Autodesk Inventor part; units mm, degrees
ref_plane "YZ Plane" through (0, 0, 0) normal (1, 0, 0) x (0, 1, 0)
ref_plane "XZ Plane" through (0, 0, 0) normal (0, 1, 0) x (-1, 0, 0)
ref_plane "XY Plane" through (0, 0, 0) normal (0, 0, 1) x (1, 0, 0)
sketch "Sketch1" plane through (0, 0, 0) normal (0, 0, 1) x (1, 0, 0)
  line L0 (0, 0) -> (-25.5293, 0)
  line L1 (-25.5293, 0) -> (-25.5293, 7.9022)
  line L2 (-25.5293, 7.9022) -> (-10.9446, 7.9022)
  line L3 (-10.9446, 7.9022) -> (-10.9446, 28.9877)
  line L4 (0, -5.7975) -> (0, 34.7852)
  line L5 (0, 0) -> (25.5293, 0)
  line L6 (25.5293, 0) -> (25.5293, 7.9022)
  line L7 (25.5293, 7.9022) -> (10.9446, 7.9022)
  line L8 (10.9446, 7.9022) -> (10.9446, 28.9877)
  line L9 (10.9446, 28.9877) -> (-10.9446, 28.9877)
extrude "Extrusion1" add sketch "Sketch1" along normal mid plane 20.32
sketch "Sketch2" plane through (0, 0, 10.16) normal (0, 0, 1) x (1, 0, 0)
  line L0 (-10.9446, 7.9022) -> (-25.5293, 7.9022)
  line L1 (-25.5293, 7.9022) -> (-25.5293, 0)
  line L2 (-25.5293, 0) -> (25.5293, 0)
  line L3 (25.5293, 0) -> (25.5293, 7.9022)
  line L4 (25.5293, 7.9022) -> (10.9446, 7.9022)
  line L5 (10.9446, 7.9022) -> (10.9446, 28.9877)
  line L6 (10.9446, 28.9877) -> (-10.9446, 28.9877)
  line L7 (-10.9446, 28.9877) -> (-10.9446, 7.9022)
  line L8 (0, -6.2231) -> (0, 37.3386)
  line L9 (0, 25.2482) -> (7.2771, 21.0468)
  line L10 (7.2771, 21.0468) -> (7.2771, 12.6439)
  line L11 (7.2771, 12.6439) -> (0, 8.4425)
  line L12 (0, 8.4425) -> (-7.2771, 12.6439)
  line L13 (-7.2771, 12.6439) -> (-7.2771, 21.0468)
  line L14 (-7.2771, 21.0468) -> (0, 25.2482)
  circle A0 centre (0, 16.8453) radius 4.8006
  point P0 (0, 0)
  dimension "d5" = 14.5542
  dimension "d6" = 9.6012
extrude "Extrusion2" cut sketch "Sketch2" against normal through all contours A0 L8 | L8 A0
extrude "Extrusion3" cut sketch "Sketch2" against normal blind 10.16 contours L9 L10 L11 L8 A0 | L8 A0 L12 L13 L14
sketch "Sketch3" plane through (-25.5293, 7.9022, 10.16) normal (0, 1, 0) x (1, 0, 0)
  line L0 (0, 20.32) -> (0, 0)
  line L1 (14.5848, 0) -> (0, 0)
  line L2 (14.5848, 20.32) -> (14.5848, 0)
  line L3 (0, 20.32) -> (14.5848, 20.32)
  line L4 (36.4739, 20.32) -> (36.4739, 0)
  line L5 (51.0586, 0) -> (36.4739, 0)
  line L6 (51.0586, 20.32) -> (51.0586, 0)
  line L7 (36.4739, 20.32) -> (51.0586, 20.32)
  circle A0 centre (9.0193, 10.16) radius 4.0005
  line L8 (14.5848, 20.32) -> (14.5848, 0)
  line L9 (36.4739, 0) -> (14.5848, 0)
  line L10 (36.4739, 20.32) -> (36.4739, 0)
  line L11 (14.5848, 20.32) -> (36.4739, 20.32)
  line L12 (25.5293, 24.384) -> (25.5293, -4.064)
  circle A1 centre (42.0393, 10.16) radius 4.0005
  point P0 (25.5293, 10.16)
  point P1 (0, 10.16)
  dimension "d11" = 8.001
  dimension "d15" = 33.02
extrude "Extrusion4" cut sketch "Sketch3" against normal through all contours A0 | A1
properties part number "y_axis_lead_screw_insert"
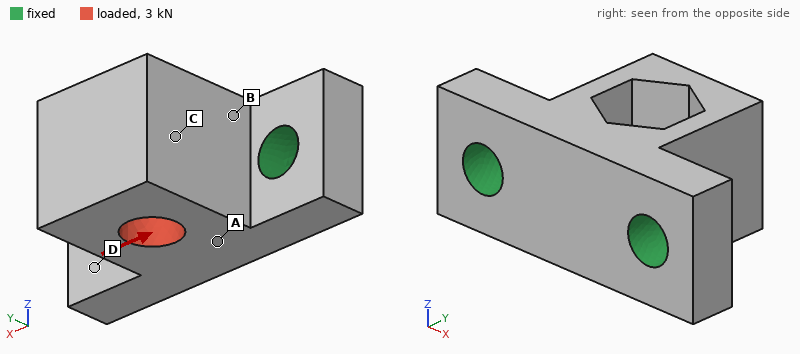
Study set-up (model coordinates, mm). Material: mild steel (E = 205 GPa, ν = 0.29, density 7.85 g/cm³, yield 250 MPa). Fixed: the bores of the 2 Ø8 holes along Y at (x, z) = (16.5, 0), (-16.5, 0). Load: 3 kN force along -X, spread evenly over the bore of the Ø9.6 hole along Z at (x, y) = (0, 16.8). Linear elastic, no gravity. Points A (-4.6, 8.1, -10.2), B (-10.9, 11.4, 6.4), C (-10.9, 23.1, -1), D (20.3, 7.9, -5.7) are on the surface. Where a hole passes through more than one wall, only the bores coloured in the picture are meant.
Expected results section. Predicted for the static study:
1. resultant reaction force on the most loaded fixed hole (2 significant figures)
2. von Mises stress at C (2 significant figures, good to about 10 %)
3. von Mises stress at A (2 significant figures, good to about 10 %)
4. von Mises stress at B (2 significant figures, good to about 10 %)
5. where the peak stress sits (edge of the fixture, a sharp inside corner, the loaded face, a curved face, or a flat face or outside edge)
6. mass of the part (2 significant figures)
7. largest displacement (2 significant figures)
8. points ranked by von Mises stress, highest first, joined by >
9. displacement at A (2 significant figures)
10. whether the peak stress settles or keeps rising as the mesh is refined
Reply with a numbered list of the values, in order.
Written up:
1. 2.1 kN
2. 12 MPa
3. 20 MPa
4. 28 MPa
5. a sharp inside corner
6. 110 g
7. 7.2 µm
8. B > A > C > D
9. 1.1 µm
10. keeps rising
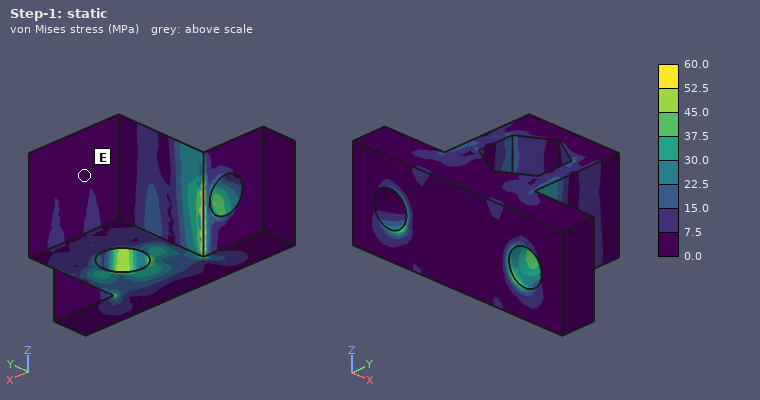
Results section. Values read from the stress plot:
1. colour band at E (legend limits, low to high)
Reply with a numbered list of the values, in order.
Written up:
1. 0.0 to 7.5 MPa
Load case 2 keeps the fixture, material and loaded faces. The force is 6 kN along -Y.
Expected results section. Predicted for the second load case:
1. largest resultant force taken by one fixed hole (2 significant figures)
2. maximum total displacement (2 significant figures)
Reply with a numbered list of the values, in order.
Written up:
1. 3.1 kN
2. 14 µm
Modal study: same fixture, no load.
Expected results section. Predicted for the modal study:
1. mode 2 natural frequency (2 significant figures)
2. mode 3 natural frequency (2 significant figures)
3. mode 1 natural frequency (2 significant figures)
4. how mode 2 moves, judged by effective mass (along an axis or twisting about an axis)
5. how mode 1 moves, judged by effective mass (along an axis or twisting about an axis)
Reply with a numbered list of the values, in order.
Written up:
1. 14 kHz
2. 22 kHz
3. 9600 Hz
4. along X
5. along Z
